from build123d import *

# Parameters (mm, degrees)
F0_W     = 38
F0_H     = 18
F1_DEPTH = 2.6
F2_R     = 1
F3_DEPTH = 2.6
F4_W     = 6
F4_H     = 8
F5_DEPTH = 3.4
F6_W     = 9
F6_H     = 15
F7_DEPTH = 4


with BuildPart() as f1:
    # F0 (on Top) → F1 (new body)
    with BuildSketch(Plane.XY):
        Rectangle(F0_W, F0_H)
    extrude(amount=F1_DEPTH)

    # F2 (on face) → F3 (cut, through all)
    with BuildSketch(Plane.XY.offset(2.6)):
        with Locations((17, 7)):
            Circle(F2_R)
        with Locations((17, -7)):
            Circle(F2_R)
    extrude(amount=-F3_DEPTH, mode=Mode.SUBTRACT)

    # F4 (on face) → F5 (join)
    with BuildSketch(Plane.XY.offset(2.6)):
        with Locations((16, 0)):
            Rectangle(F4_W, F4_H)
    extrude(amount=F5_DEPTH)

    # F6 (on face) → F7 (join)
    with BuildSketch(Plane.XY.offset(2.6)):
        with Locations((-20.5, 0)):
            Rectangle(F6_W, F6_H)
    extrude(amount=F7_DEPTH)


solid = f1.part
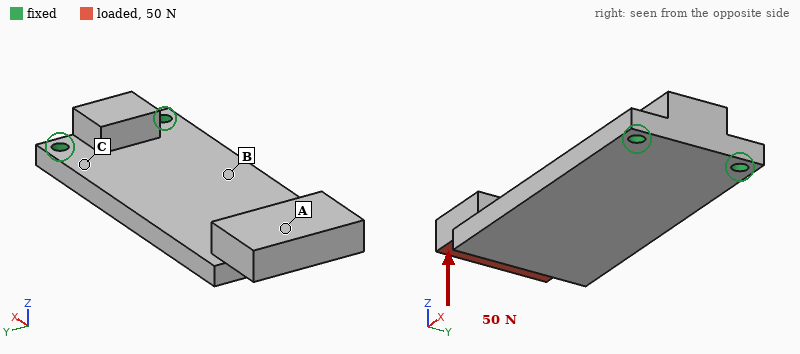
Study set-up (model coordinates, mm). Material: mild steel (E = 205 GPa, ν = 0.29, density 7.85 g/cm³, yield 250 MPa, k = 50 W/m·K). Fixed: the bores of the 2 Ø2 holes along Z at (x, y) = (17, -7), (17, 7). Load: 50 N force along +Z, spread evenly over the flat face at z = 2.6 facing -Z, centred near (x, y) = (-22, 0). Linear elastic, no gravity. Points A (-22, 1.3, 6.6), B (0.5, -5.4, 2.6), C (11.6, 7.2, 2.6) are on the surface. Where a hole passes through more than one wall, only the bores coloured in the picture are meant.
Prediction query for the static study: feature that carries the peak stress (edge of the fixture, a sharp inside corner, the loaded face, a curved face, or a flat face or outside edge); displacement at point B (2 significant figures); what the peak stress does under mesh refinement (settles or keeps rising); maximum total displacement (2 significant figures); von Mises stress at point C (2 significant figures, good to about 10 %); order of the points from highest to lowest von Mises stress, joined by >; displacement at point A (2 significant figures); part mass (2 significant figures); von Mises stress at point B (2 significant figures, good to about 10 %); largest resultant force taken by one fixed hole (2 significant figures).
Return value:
edge of the fixture
0.044 mm
keeps rising
0.21 mm
82 MPa
C > B > A
0.19 mm
19 g
55 MPa
26 N
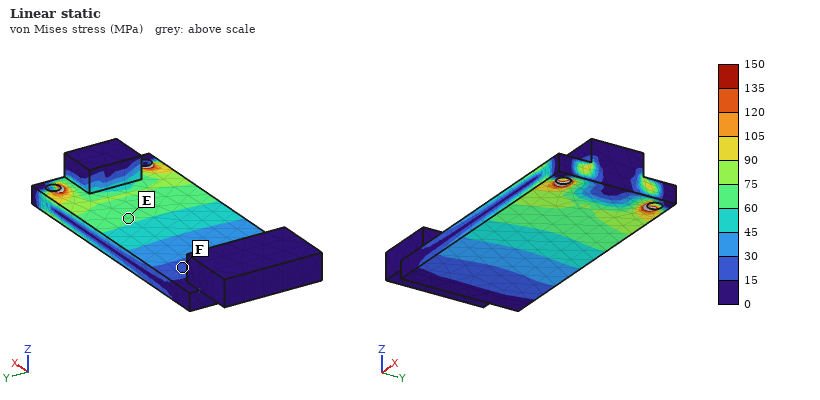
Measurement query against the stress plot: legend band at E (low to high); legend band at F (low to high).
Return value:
60 to 75 MPa
15 to 30 MPa
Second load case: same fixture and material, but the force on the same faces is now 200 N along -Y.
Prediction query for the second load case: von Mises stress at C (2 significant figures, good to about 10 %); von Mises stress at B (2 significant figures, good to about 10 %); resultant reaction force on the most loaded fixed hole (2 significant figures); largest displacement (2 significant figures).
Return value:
37 MPa
27 MPa
550 N
25 µm
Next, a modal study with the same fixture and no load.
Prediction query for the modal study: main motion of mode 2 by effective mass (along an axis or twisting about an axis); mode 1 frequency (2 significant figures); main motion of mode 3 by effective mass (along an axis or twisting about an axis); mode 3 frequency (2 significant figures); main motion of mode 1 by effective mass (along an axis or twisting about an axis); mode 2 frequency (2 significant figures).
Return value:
along Y
1000 Hz
along Z
6700 Hz
along Z
4900 Hz
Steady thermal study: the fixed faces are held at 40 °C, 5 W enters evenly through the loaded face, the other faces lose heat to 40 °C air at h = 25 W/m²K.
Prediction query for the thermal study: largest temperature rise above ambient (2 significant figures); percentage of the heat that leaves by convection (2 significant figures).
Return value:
67 K
32 %
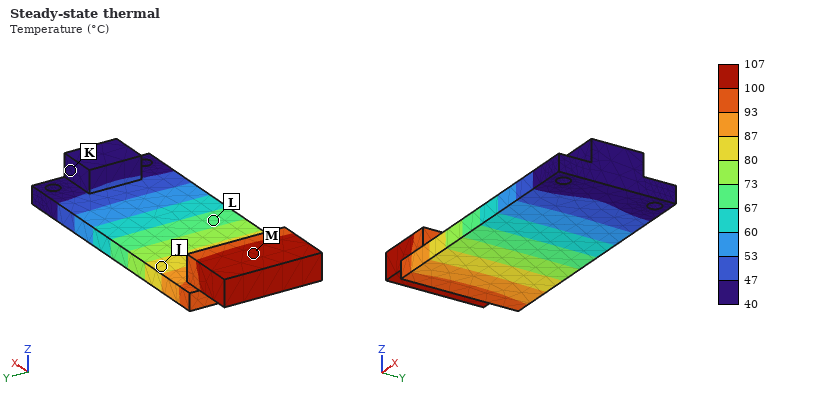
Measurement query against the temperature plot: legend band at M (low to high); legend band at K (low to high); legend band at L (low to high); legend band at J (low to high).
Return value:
100 to 107 °C
40 to 47 °C
67 to 73 °C
80 to 87 °C
